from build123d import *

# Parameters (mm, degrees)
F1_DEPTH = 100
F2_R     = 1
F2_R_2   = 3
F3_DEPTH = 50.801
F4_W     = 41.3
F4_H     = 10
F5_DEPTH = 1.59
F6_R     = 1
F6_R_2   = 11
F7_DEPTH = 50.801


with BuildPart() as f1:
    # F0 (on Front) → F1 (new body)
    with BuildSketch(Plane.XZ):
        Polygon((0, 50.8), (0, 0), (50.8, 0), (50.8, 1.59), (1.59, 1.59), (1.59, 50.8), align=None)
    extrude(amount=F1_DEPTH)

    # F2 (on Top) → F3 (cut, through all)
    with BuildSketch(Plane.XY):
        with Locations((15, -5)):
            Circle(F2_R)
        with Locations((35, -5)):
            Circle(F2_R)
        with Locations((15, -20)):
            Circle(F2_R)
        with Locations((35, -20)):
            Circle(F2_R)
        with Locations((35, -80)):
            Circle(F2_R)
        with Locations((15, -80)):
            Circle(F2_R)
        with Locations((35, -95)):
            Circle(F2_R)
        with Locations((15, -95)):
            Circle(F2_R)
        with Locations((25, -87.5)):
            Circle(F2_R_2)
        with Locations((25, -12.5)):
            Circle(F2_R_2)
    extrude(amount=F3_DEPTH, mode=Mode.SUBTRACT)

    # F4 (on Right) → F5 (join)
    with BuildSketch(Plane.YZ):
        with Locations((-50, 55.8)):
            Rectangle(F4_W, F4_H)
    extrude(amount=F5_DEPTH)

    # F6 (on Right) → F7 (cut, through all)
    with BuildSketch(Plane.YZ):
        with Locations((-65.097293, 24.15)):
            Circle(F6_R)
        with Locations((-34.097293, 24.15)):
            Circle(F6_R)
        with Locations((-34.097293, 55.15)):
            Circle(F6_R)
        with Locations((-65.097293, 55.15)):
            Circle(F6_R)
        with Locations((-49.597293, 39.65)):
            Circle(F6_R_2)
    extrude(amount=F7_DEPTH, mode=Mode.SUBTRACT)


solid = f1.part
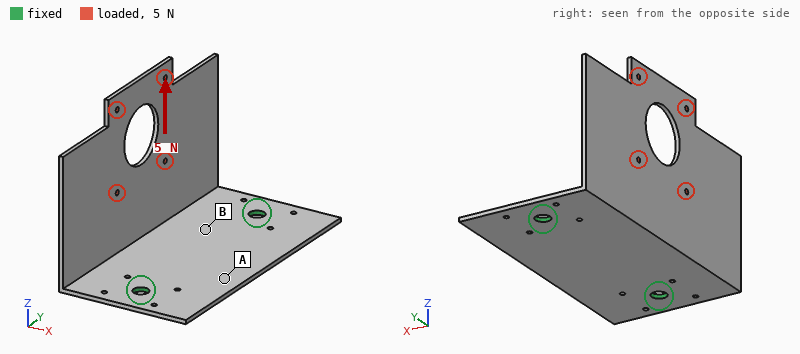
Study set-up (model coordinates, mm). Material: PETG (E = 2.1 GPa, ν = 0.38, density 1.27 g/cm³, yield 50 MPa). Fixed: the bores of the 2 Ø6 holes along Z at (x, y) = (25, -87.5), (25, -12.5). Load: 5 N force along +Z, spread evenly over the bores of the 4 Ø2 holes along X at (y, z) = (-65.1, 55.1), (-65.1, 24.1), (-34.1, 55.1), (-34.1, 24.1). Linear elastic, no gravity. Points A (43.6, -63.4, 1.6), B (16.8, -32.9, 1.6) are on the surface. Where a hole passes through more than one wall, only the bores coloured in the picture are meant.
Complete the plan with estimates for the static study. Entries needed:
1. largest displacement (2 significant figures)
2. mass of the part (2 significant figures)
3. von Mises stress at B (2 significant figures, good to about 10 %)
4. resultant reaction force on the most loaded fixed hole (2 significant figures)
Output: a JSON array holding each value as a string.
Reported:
["1.4 mm", "20 g", "1.1 MPa", "2.5 N"]
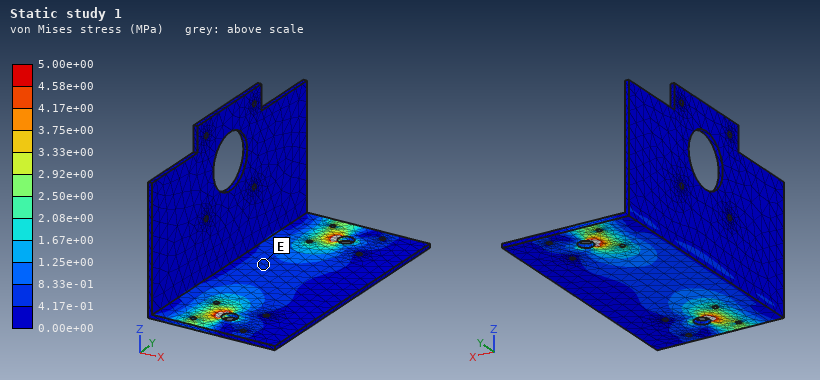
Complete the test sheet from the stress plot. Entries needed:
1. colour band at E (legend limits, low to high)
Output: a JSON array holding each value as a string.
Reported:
["4.17e-01 to 8.33e-01 MPa"]
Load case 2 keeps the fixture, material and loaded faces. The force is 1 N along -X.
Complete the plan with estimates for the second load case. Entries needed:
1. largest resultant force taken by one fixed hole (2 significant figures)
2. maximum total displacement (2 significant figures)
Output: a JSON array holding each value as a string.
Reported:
["0.52 N", "1.4 mm"]
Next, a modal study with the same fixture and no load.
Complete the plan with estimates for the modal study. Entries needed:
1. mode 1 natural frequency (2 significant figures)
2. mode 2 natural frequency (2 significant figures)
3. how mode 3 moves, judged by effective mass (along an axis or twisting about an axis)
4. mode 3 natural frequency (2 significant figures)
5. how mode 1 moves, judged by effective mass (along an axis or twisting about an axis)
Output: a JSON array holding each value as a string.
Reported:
["69 Hz", "140 Hz", "along Z", "230 Hz", "along X"]
